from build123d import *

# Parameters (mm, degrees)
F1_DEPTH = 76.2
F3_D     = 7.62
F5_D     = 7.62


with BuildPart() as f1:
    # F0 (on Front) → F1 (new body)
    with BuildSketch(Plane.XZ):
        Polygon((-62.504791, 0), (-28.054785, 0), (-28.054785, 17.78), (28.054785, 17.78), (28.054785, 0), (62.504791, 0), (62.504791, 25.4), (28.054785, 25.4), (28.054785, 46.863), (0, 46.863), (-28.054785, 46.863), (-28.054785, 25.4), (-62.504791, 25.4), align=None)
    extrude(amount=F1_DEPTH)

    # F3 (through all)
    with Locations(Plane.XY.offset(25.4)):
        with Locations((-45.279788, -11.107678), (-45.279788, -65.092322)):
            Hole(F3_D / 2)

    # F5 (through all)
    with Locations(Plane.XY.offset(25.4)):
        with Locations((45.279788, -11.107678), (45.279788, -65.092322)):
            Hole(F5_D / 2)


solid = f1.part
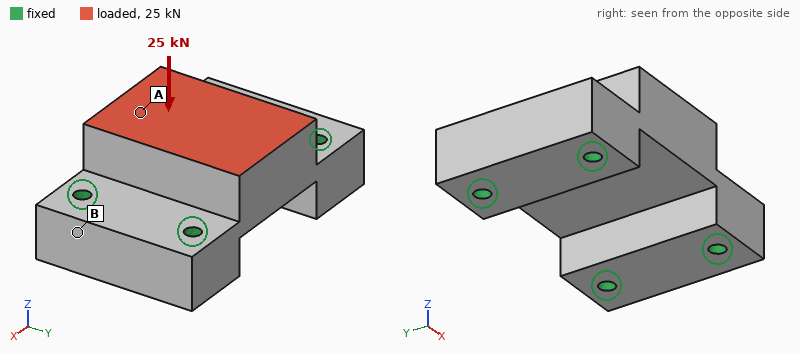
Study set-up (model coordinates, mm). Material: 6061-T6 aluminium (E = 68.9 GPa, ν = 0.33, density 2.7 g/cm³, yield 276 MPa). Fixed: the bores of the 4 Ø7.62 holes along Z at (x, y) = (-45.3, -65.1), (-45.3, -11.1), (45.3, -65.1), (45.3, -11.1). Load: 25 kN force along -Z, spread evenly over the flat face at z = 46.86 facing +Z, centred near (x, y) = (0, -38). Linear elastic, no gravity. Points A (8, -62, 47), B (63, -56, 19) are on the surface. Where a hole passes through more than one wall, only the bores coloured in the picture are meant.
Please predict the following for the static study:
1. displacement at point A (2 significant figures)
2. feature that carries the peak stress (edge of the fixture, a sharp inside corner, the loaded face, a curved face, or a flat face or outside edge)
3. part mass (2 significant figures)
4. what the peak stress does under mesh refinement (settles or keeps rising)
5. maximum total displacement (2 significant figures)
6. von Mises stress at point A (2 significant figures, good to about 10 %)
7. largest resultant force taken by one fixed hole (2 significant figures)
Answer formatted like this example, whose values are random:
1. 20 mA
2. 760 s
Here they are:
1. 20 µm
2. edge of the fixture
3. 680 g
4. keeps rising
5. 22 µm
6. 8.1 MPa
7. 7.7 kN
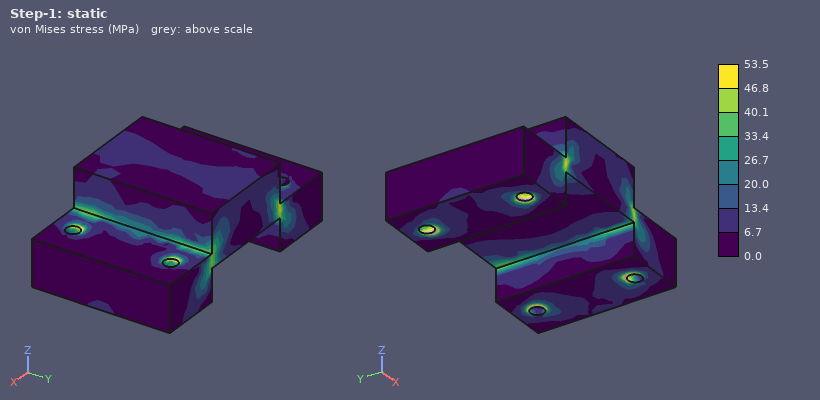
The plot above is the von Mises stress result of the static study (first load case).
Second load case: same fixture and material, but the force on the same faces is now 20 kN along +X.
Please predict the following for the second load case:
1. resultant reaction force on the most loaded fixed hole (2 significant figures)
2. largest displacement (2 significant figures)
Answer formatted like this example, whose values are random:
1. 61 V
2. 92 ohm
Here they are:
1. 6.6 kN
2. 20 µm
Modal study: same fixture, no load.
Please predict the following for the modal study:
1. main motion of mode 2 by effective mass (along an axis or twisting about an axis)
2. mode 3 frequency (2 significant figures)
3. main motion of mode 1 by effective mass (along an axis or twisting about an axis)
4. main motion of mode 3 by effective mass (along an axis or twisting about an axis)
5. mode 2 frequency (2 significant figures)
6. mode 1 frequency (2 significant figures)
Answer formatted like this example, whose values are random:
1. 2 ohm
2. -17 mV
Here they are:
1. along Z
2. 13 kHz
3. along Y
4. along Y
5. 9600 Hz
6. 8200 Hz
